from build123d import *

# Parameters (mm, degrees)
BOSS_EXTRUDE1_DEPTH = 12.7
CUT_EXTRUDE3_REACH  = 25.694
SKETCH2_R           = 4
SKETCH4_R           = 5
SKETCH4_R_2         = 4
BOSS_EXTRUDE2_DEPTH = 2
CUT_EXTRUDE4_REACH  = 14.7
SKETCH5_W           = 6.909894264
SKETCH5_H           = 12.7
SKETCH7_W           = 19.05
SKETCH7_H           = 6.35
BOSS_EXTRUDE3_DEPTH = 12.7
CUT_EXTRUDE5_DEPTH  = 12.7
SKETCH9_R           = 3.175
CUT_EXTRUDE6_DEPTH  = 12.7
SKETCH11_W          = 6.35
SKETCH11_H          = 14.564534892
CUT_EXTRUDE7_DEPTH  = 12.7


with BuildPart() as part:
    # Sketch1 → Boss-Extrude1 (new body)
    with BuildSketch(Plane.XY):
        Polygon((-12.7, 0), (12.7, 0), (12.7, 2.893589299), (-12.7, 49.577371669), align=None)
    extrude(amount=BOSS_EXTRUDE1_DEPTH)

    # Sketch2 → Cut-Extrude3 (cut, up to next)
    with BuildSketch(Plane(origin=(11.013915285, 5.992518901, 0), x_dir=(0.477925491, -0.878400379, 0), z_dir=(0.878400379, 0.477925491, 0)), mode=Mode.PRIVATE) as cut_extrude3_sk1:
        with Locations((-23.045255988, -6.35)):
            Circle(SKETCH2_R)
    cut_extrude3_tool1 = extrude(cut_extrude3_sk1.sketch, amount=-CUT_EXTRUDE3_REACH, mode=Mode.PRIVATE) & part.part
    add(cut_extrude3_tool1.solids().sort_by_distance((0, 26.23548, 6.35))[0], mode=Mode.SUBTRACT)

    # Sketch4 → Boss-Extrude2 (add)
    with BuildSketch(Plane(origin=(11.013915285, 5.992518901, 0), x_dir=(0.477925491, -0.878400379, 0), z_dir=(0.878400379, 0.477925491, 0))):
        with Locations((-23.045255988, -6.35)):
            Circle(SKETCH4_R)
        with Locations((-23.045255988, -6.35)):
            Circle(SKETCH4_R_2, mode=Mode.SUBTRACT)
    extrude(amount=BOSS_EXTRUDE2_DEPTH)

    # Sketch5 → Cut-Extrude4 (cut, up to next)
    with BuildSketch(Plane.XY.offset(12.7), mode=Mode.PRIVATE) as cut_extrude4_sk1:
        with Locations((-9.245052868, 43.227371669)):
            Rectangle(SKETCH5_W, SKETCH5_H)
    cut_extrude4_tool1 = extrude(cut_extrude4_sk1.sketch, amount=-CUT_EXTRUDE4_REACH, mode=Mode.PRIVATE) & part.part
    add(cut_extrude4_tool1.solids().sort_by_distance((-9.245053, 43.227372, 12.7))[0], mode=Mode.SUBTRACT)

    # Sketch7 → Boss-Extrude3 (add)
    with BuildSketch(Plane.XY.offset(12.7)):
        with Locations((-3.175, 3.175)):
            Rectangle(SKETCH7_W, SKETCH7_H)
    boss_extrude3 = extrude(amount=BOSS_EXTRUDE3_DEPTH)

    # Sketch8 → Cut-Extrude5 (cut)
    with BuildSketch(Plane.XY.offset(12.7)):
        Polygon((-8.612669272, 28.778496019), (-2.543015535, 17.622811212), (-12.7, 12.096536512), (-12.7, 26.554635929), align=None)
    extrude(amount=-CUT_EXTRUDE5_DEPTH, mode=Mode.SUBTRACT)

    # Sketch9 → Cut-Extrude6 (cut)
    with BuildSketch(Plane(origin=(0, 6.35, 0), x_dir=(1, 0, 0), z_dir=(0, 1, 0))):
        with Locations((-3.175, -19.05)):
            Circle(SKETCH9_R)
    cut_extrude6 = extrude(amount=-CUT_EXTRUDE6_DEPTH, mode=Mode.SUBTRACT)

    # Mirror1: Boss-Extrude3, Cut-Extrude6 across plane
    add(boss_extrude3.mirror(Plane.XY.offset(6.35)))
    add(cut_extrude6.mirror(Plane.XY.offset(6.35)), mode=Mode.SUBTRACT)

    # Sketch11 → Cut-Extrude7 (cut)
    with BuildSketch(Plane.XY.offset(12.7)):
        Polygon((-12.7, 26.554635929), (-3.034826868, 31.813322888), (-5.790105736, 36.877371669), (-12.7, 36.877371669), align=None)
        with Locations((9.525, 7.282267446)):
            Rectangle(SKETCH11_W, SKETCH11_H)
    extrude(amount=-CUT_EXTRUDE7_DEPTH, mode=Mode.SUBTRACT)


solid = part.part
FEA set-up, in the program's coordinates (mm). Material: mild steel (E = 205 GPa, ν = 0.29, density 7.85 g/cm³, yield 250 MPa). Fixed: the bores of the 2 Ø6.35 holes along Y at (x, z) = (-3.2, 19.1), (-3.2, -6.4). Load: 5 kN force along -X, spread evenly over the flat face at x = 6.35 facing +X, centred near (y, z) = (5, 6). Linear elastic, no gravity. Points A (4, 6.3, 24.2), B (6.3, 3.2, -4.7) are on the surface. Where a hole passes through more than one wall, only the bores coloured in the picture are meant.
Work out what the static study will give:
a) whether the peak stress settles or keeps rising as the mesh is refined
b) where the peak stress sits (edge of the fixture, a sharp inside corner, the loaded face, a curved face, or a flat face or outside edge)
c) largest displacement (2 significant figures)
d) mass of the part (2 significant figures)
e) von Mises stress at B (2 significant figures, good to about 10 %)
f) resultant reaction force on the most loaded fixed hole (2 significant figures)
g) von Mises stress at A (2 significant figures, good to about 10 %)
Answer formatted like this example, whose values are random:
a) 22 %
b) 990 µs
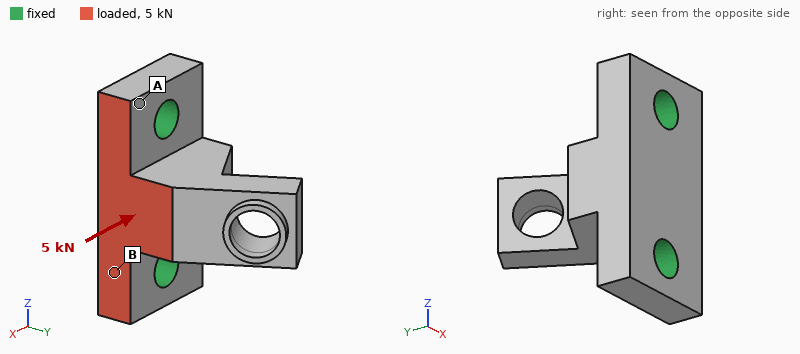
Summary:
a) keeps rising
b) edge of the fixture
c) 10 µm
d) 58 g
e) 28 MPa
f) 2.5 kN
g) 14 MPa
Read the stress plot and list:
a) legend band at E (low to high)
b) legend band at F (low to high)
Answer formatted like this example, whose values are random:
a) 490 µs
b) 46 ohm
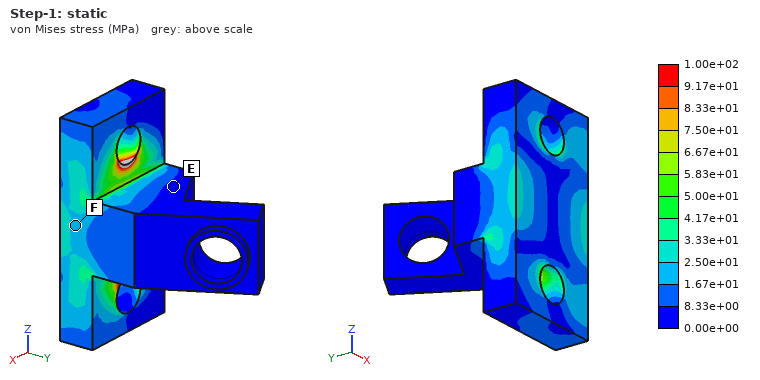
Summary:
a) 0.00e+00 to 8.33e+00 MPa
b) 1.67e+01 to 2.50e+01 MPa
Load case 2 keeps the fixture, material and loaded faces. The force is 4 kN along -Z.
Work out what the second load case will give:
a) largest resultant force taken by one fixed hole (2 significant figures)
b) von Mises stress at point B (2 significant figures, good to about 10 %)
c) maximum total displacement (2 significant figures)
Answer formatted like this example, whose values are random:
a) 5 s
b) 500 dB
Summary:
a) 2.4 kN
b) 22 MPa
c) 4.0 µm
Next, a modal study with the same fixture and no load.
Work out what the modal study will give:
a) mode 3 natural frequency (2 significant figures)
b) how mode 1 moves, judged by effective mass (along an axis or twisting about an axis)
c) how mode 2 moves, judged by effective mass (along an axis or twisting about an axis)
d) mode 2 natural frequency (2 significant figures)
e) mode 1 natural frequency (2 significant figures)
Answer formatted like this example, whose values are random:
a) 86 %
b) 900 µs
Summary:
a) 23 kHz
b) along X
c) along Z
d) 14 kHz
e) 11 kHz
